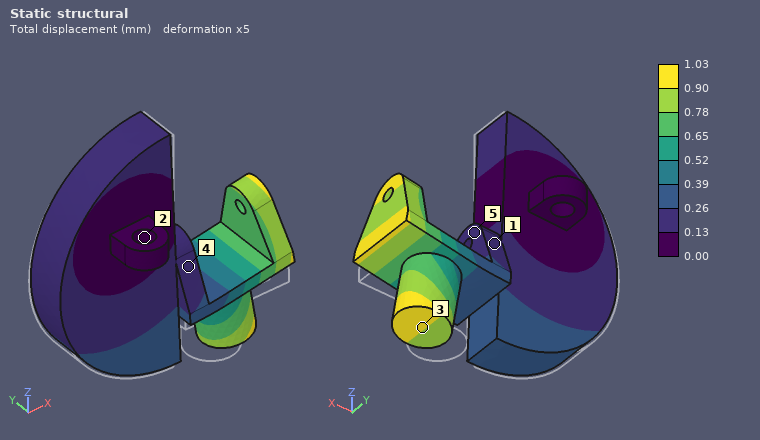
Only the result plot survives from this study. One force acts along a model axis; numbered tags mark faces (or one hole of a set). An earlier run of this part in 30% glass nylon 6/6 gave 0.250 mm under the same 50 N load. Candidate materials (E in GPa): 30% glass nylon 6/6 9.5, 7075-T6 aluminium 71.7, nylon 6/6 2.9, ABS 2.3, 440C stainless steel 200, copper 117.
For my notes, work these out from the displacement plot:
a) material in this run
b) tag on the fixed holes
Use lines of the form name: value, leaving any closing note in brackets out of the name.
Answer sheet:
material in this run: ABS
tag on the fixed holes: 2
